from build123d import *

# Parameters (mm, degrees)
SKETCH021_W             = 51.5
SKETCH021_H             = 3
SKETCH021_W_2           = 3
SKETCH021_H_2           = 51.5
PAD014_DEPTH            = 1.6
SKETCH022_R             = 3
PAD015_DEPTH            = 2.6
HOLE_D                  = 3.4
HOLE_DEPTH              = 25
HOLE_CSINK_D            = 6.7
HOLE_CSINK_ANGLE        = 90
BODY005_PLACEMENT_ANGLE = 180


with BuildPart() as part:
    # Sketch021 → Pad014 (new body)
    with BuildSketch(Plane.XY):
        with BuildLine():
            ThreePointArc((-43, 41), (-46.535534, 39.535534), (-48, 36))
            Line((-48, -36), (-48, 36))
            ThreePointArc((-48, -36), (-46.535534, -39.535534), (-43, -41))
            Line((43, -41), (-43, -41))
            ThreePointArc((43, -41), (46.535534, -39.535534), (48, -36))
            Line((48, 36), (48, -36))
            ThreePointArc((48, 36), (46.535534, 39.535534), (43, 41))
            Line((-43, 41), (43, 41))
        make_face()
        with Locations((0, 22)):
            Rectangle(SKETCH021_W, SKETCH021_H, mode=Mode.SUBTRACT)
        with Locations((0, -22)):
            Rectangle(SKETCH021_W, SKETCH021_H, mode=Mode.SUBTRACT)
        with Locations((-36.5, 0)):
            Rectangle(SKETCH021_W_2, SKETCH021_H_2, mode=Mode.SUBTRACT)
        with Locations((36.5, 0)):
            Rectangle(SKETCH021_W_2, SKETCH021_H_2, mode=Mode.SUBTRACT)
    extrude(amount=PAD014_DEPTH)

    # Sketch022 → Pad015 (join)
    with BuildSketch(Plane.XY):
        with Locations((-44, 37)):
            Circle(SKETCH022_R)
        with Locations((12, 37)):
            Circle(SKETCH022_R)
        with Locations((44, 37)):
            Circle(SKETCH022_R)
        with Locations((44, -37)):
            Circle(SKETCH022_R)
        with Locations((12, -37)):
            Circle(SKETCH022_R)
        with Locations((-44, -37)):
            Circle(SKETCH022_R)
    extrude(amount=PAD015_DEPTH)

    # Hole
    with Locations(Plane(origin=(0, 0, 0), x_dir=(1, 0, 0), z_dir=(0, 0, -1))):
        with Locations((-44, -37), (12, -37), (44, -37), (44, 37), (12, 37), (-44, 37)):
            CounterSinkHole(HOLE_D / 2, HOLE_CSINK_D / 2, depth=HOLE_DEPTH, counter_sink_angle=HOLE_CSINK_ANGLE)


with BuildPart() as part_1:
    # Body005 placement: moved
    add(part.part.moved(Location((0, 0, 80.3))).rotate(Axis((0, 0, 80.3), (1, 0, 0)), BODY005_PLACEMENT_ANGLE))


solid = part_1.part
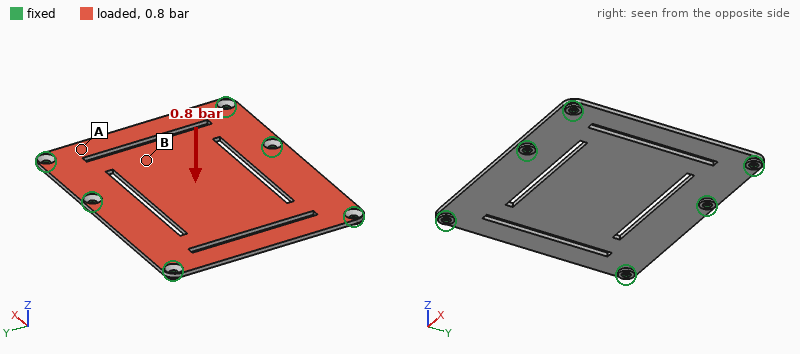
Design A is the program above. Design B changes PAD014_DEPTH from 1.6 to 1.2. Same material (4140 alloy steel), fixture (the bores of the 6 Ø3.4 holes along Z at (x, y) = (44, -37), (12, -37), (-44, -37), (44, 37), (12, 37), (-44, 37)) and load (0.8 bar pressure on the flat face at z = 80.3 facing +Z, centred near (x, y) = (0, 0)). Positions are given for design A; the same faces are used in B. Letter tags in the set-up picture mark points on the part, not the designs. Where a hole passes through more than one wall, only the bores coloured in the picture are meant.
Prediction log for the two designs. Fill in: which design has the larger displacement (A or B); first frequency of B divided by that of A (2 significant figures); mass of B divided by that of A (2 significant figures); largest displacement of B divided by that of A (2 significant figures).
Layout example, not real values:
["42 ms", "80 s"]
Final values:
["B", "0.77", "0.75", "2.2"]
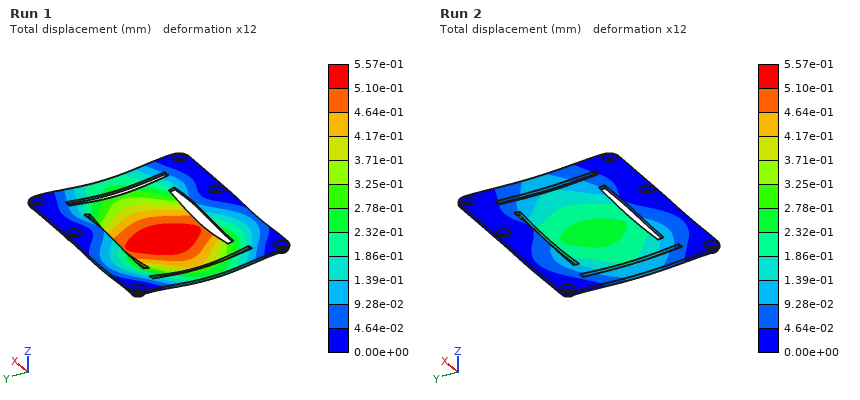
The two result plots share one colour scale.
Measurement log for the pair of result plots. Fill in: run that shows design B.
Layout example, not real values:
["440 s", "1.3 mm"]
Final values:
["Run 1"]
